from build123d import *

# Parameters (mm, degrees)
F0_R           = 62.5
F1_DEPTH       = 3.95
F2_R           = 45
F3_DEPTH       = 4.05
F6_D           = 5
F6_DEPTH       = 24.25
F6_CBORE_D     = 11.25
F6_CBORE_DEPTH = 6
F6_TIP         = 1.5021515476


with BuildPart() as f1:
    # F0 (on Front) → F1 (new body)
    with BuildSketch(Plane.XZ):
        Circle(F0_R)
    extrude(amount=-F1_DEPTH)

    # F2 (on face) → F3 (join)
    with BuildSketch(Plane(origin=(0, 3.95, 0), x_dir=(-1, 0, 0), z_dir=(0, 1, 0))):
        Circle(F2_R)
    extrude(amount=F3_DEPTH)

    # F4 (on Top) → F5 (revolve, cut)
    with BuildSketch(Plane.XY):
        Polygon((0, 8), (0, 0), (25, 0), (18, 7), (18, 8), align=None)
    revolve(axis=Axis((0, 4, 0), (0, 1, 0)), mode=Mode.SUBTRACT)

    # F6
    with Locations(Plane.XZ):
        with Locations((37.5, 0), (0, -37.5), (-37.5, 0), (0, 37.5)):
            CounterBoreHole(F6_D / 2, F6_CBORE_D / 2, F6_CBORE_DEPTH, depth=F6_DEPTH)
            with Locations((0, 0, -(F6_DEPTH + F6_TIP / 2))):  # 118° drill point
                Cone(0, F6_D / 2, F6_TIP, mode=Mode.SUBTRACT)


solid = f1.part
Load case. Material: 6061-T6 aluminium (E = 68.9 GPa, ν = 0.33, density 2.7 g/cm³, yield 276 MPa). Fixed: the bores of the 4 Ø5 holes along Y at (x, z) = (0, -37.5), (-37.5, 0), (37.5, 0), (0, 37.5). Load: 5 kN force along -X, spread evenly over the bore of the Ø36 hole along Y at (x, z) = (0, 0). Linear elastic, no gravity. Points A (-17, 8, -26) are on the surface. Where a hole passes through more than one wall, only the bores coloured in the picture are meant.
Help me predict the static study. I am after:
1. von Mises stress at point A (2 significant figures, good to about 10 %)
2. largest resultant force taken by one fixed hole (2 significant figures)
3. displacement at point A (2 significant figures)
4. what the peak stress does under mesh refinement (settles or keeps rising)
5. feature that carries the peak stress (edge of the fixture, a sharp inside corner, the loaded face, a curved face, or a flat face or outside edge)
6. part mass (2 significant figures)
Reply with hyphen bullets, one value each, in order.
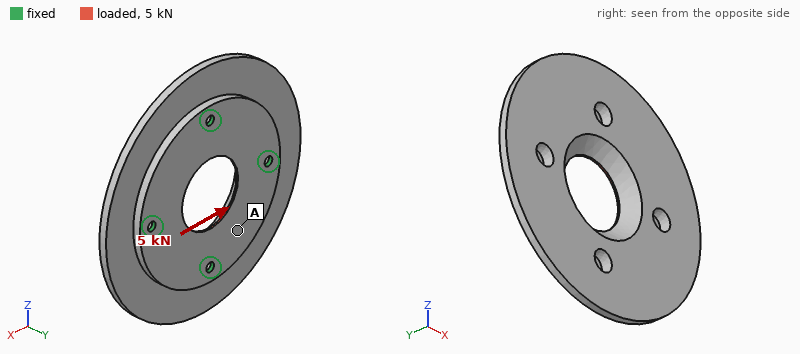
- 6.4 MPa
- 1.3 kN
- 4.8 µm
- keeps rising
- edge of the fixture
- 160 g
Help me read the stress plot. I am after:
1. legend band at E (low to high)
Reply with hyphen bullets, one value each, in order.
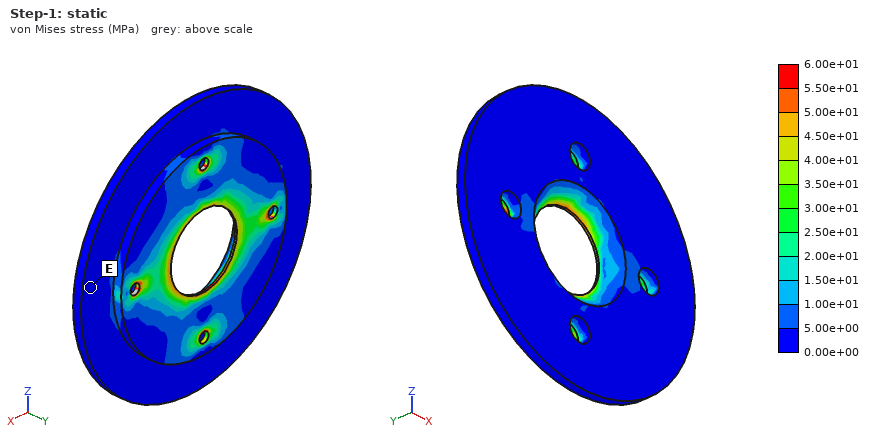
- 0.00e+00 to 5.00e+00 MPa
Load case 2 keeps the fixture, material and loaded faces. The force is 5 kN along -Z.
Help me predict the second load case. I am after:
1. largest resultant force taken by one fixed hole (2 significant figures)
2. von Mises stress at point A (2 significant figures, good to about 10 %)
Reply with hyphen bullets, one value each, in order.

- 1.3 kN
- 7.0 MPa
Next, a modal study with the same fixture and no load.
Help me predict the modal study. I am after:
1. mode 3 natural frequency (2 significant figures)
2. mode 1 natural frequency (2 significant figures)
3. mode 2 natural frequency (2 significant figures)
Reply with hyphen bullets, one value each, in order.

- 3800 Hz
- 3000 Hz
- 3700 Hz
